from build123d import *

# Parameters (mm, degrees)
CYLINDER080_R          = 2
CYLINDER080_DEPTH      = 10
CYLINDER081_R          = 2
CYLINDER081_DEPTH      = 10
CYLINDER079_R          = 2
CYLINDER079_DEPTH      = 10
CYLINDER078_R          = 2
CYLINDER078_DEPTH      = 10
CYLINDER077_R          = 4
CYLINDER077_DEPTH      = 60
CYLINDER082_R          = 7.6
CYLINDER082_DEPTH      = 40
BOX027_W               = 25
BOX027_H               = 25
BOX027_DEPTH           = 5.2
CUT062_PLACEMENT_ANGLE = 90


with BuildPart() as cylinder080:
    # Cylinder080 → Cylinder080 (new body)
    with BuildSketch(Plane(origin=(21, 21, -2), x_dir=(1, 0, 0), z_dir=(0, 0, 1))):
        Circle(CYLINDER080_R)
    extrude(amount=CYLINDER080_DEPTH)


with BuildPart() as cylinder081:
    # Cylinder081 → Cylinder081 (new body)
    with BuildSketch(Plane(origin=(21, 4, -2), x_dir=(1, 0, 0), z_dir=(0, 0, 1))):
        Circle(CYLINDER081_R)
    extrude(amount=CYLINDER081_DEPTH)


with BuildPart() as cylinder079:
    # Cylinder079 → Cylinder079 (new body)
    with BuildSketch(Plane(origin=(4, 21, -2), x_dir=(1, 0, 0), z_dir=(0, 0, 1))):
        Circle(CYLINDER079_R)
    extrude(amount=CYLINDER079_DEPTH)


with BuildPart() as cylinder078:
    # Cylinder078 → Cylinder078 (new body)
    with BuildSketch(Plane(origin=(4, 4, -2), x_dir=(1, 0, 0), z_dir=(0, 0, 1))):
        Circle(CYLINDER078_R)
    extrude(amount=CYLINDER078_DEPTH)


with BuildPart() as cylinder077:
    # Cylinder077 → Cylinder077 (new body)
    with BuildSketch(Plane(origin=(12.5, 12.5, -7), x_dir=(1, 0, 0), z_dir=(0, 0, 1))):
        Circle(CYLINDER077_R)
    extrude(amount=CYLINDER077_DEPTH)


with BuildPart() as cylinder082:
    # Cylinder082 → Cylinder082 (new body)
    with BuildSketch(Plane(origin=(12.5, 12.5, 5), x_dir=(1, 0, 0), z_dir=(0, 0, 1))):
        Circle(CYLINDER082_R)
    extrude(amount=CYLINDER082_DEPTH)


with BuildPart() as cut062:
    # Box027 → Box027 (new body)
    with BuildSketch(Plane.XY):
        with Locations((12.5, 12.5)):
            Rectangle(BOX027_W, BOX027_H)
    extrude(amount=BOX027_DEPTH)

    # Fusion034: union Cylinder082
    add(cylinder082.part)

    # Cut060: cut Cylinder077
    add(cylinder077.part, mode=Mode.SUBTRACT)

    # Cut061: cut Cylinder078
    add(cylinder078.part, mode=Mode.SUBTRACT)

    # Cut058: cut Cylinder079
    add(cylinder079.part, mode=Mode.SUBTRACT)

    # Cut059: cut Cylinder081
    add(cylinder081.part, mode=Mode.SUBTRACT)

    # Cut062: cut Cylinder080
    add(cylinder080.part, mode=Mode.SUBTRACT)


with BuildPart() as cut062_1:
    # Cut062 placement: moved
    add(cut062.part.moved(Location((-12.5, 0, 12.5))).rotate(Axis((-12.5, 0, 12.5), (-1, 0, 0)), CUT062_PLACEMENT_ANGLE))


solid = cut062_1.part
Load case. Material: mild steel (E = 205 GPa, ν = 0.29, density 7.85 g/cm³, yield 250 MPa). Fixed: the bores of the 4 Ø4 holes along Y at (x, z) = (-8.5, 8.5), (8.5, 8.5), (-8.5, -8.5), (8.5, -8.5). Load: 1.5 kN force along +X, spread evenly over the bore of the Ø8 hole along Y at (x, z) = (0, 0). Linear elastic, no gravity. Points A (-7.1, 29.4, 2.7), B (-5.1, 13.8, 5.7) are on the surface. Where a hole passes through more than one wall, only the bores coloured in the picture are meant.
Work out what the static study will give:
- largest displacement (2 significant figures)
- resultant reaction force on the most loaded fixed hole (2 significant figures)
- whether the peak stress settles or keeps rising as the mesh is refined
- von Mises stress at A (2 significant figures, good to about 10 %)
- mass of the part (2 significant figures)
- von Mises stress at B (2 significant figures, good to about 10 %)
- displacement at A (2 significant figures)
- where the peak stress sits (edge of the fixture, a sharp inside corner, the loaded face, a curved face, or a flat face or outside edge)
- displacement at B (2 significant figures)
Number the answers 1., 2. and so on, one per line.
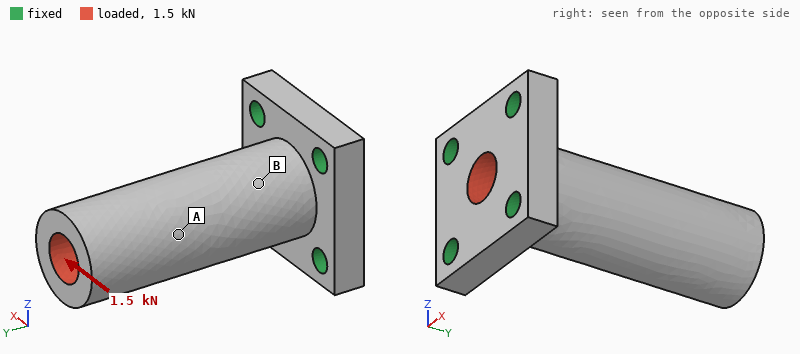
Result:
1. 40 µm
2. 1.1 kN
3. keeps rising
4. 12 MPa
5. 62 g
6. 36 MPa
7. 24 µm
8. edge of the fixture
9. 7.7 µm
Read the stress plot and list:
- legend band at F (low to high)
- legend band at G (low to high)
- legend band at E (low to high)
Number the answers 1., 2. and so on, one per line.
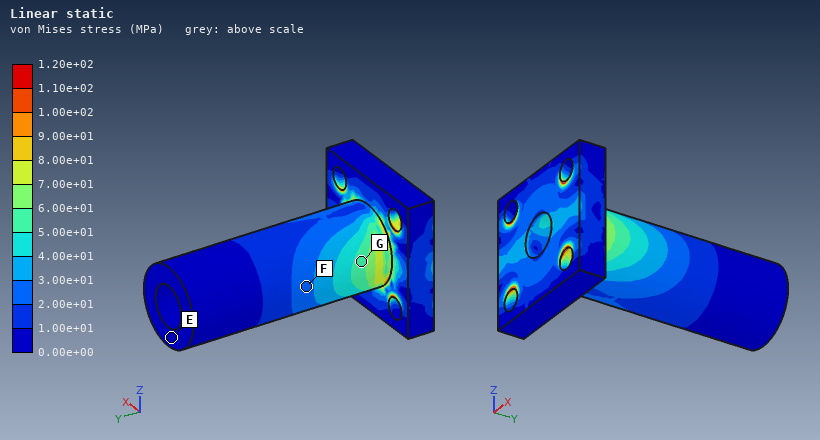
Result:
1. 2.00e+01 to 3.00e+01 MPa
2. 5.00e+01 to 6.00e+01 MPa
3. 0.00e+00 to 1.00e+01 MPa
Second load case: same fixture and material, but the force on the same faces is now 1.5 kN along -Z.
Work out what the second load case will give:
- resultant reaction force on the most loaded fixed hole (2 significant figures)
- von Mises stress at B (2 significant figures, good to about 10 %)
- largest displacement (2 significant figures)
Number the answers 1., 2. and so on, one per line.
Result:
1. 1.1 kN
2. 39 MPa
3. 40 µm
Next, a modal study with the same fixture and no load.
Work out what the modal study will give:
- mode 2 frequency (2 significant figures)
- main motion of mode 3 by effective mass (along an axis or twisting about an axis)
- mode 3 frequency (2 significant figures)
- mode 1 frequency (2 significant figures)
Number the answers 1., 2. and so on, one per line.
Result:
1. 5500 Hz
2. twisting about Y
3. 19 kHz
4. 5500 Hz
